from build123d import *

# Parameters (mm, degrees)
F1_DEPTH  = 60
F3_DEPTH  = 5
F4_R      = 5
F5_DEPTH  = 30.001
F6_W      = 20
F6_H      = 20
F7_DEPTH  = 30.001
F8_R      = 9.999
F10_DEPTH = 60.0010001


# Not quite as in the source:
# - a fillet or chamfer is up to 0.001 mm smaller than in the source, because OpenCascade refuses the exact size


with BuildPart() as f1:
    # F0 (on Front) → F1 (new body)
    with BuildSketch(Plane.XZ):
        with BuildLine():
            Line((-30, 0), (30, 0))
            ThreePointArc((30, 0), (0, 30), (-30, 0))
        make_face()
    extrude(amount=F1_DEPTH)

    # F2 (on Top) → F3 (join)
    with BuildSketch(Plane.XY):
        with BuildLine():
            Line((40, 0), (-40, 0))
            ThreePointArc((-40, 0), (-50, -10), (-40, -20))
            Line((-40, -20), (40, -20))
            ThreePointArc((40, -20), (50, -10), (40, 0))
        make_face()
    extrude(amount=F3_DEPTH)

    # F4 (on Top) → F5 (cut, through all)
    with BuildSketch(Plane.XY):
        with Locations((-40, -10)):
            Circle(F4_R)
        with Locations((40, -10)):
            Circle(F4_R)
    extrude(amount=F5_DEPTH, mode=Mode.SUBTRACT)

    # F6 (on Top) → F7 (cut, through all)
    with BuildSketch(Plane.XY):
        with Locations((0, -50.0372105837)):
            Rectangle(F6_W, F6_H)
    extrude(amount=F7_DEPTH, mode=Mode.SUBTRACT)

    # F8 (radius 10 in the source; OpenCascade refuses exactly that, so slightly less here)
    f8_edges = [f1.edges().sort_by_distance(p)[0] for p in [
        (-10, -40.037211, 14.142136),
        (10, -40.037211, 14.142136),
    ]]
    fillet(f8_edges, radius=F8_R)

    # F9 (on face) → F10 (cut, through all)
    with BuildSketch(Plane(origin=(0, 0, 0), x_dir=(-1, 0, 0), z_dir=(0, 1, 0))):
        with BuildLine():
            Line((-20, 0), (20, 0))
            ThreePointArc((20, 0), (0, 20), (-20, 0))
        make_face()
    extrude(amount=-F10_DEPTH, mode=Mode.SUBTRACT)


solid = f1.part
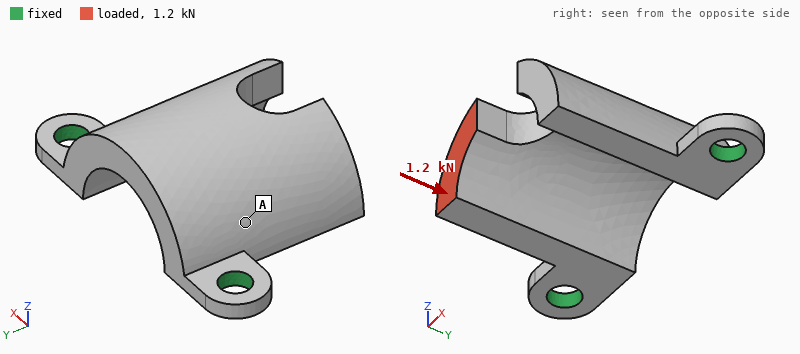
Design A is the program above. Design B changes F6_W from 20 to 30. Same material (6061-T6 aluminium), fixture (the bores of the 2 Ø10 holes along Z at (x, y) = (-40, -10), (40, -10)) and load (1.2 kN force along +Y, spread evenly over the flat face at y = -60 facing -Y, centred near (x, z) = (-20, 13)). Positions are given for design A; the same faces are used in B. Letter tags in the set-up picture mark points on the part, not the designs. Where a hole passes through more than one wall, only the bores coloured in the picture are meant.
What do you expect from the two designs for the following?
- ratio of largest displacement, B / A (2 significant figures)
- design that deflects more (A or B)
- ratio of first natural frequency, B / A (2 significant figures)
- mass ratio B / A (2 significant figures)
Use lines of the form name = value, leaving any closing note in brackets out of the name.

ratio of largest displacement, B / A = 0.80
design that deflects more = A
ratio of first natural frequency, B / A = 1.1
mass ratio B / A = 0.95
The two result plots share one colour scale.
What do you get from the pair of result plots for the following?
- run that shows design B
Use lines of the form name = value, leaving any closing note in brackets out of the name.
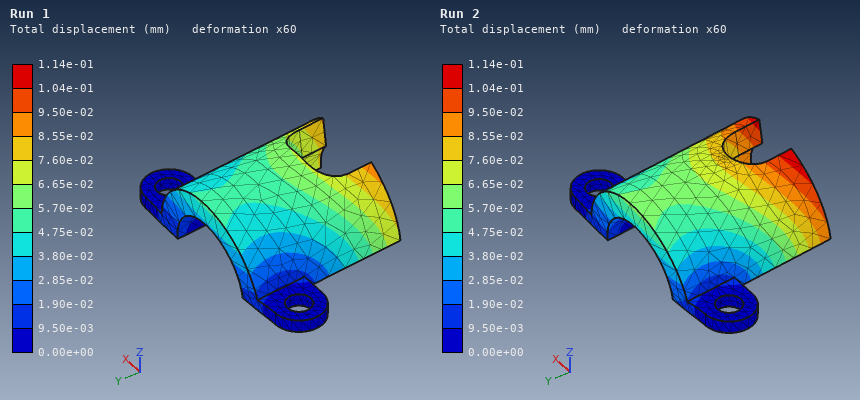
run that shows design B = Run 1
